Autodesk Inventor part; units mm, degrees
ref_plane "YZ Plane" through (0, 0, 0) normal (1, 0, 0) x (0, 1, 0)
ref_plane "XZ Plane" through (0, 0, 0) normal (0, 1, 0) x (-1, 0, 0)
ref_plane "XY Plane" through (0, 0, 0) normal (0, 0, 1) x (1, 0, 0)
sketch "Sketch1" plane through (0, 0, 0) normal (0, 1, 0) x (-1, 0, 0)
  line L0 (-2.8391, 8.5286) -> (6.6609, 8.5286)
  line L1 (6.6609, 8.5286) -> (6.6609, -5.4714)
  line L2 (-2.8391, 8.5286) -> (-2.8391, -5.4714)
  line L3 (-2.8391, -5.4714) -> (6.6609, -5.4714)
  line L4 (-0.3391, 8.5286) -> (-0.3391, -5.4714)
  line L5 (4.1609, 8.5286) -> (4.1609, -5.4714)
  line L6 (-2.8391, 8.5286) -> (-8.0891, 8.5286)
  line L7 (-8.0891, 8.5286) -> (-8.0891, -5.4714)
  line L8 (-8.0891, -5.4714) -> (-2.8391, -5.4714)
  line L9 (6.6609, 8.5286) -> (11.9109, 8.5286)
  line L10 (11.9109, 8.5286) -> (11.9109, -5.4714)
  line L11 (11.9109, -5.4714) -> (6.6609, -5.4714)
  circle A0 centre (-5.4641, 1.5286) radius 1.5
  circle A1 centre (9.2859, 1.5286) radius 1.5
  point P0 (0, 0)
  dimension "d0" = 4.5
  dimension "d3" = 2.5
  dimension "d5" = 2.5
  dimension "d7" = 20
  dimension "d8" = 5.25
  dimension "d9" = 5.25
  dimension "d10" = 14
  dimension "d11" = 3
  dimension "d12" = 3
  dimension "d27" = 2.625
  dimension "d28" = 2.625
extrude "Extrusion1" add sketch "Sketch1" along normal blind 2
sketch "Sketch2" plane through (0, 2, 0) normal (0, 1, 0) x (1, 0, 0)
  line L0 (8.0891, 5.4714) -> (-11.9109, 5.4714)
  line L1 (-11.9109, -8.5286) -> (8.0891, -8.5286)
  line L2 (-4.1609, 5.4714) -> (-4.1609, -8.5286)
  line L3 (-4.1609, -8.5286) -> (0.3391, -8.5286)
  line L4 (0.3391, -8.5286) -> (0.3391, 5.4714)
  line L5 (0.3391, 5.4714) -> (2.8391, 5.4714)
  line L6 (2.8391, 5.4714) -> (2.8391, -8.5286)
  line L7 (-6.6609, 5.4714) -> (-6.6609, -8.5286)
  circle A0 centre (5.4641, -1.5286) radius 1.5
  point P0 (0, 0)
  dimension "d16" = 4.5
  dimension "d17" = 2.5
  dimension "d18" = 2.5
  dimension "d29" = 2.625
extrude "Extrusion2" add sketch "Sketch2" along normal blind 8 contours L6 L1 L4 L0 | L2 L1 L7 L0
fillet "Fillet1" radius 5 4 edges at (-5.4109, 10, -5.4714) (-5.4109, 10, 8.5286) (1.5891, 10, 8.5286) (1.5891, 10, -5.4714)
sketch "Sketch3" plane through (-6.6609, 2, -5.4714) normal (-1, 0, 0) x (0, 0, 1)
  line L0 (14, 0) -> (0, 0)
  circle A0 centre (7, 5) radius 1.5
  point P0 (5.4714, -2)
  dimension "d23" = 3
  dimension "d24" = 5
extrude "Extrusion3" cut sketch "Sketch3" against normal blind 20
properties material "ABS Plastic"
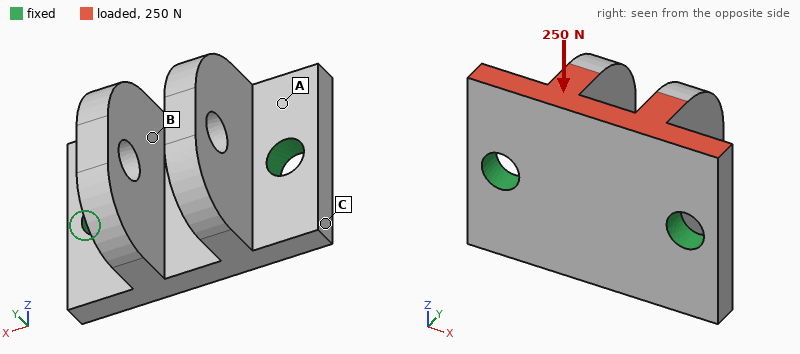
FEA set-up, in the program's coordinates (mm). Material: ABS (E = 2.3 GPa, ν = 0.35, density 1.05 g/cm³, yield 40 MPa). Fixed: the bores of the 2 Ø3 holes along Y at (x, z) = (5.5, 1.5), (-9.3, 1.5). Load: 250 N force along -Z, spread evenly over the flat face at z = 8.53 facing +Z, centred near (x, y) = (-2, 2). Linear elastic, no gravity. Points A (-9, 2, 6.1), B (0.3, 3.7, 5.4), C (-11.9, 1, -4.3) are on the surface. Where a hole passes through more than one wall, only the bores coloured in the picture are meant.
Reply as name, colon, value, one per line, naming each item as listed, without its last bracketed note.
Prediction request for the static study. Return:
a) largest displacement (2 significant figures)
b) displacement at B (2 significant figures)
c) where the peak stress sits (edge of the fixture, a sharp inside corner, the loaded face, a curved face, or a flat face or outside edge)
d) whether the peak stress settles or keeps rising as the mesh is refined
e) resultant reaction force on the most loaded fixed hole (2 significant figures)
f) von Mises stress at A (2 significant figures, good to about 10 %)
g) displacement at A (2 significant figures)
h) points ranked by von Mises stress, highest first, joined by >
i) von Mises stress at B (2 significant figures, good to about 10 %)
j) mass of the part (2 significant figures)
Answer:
largest displacement: 79 µm
displacement at B: 46 µm
where the peak stress sits: edge of the fixture
whether the peak stress settles or keeps rising as the mesh is refined: keeps rising
resultant reaction force on the most loaded fixed hole: 130 N
von Mises stress at A: 7.5 MPa
displacement at A: 24 µm
points ranked by von Mises stress, highest first, joined by >: A > B > C
von Mises stress at B: 3.5 MPa
mass of the part: 1.1 g
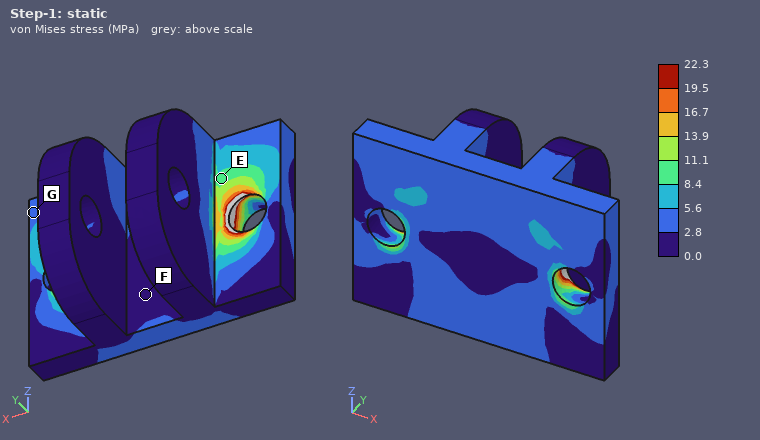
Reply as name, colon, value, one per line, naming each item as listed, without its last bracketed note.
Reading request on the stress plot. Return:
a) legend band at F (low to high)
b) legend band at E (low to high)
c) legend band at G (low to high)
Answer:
legend band at F: 0.0 to 2.8 MPa
legend band at E: 8.4 to 11.1 MPa
legend band at G: 2.8 to 5.6 MPa
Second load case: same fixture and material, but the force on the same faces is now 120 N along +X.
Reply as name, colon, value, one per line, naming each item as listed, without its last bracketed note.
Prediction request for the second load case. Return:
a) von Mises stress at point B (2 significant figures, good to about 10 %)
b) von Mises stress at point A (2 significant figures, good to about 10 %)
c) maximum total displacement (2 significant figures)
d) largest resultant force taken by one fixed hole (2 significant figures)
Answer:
von Mises stress at point B: 2.7 MPa
von Mises stress at point A: 5.0 MPa
maximum total displacement: 47 µm
largest resultant force taken by one fixed hole: 77 N
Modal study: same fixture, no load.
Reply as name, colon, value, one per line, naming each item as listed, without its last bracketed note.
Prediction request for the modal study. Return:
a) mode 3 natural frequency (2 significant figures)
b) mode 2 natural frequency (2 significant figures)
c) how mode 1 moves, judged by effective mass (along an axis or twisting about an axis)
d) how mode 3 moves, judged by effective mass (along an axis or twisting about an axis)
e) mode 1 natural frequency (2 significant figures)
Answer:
mode 3 natural frequency: 7900 Hz
mode 2 natural frequency: 5400 Hz
how mode 1 moves, judged by effective mass: along Z
how mode 3 moves, judged by effective mass: along X
mode 1 natural frequency: 4800 Hz
